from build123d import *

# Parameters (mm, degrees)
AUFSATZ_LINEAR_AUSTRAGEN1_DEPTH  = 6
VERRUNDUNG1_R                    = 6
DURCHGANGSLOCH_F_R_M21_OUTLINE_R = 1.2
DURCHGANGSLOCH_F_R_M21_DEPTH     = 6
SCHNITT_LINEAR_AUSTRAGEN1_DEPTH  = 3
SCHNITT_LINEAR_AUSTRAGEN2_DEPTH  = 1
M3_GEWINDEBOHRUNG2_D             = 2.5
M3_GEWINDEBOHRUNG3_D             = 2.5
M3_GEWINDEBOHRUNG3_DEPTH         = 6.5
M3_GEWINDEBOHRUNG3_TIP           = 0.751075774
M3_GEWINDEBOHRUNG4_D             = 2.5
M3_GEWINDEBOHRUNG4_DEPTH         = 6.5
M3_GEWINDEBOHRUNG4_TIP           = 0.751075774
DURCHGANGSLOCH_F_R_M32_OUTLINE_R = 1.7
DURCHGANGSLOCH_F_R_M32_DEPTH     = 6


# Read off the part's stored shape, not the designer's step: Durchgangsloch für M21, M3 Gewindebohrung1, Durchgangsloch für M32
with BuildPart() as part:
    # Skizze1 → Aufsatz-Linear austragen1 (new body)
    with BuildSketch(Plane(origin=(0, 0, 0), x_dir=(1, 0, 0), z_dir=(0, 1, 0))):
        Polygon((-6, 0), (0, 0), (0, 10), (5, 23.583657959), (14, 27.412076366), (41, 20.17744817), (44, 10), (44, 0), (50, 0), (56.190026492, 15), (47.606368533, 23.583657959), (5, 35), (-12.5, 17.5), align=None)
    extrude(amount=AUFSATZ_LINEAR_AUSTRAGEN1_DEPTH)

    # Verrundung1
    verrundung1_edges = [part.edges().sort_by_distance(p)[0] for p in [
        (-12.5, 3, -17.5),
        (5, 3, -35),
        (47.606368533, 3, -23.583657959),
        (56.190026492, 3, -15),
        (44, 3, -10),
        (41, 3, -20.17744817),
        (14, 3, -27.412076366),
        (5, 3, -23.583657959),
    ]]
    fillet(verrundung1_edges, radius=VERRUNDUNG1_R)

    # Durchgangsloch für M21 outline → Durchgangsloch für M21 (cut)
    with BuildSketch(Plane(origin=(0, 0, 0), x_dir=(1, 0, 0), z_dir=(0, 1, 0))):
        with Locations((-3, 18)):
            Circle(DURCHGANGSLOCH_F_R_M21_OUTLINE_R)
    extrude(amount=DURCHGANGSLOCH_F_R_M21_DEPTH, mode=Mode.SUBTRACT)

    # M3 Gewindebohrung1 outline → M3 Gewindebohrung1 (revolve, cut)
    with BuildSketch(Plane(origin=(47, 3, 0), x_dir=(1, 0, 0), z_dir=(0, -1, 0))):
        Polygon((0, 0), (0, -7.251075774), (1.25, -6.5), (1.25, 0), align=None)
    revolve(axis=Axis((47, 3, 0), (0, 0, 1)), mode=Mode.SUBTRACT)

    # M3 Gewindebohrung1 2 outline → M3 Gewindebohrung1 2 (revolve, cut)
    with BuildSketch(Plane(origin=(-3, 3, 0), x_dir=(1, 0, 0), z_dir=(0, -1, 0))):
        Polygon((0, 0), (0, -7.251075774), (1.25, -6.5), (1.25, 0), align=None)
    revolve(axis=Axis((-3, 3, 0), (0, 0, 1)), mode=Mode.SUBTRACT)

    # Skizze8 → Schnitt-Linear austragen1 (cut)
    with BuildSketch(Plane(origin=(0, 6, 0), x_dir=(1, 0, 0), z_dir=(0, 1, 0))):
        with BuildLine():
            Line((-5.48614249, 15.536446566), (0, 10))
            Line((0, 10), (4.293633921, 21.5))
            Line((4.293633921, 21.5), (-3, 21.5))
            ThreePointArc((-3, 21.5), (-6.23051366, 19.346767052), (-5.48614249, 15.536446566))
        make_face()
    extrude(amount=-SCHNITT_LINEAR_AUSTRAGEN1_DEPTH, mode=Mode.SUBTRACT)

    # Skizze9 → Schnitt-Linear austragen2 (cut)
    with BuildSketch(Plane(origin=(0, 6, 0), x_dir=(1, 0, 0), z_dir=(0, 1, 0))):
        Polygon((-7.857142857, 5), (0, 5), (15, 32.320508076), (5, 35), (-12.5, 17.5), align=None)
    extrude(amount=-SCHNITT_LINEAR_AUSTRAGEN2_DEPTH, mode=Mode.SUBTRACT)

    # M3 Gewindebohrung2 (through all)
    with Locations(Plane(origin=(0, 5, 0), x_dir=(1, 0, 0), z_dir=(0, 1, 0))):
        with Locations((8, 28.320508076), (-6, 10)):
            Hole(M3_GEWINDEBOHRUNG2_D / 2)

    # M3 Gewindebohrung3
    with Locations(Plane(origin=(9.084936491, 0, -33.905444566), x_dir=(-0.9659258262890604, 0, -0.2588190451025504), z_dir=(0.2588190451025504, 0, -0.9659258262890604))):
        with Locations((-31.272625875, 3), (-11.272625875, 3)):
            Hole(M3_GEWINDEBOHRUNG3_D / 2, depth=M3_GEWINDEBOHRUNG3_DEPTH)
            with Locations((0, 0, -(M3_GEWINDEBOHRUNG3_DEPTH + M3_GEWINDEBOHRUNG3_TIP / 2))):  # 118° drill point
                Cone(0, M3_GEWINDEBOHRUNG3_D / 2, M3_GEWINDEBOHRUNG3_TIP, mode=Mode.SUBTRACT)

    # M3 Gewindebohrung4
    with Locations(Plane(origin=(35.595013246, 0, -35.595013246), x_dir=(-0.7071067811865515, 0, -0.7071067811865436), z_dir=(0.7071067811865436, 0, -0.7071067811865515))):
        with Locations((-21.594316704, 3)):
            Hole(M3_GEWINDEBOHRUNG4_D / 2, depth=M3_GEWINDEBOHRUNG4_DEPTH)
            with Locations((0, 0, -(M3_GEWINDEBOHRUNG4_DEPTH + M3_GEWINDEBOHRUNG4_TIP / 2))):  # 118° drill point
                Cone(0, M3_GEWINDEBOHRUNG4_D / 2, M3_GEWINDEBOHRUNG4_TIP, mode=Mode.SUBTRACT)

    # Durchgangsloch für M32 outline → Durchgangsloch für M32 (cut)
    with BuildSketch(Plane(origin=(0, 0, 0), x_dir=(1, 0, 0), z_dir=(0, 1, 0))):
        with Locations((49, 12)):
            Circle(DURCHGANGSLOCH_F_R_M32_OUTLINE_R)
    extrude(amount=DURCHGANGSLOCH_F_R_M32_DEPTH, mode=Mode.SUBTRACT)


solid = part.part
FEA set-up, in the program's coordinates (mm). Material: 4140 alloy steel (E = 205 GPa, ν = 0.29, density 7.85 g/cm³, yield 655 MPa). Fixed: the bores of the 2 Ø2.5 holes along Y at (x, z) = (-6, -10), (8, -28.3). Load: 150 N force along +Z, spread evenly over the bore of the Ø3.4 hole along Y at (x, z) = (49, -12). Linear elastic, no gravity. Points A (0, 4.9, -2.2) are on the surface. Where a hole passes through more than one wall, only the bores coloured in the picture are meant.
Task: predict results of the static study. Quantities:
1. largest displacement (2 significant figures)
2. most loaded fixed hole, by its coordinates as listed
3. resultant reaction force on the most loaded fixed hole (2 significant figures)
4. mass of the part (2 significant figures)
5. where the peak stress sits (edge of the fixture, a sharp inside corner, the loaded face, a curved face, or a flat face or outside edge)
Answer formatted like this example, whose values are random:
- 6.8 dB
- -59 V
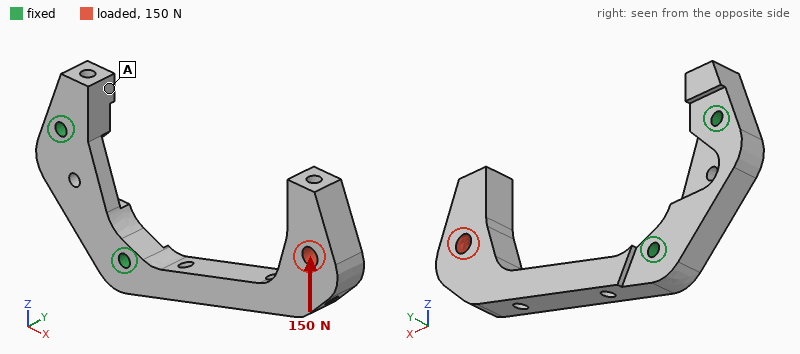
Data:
- 0.39 mm
- (8, -28.3)
- 410 N
- 30 g
- a curved face
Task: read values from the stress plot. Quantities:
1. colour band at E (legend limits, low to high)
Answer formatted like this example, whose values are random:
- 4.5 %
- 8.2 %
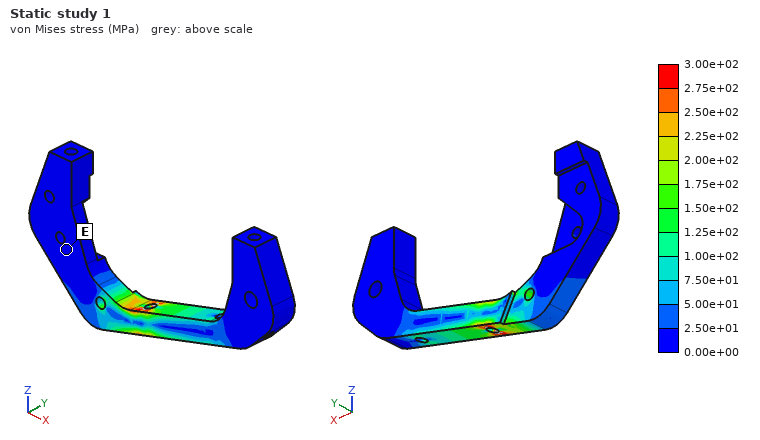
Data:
- 0.00e+00 to 2.50e+01 MPa
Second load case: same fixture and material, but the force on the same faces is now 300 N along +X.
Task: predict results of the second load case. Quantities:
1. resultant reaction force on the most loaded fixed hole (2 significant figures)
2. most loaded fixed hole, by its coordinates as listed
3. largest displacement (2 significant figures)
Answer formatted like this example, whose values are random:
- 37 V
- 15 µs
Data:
- 390 N
- (8, -28.3)
- 0.48 mm
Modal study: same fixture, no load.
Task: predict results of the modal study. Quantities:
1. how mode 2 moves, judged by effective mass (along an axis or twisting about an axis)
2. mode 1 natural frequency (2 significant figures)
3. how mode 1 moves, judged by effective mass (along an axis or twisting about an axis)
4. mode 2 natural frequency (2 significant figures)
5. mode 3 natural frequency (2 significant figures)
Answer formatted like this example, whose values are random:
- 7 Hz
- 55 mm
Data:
- along Y
- 1000 Hz
- along Z
- 1100 Hz
- 4100 Hz
